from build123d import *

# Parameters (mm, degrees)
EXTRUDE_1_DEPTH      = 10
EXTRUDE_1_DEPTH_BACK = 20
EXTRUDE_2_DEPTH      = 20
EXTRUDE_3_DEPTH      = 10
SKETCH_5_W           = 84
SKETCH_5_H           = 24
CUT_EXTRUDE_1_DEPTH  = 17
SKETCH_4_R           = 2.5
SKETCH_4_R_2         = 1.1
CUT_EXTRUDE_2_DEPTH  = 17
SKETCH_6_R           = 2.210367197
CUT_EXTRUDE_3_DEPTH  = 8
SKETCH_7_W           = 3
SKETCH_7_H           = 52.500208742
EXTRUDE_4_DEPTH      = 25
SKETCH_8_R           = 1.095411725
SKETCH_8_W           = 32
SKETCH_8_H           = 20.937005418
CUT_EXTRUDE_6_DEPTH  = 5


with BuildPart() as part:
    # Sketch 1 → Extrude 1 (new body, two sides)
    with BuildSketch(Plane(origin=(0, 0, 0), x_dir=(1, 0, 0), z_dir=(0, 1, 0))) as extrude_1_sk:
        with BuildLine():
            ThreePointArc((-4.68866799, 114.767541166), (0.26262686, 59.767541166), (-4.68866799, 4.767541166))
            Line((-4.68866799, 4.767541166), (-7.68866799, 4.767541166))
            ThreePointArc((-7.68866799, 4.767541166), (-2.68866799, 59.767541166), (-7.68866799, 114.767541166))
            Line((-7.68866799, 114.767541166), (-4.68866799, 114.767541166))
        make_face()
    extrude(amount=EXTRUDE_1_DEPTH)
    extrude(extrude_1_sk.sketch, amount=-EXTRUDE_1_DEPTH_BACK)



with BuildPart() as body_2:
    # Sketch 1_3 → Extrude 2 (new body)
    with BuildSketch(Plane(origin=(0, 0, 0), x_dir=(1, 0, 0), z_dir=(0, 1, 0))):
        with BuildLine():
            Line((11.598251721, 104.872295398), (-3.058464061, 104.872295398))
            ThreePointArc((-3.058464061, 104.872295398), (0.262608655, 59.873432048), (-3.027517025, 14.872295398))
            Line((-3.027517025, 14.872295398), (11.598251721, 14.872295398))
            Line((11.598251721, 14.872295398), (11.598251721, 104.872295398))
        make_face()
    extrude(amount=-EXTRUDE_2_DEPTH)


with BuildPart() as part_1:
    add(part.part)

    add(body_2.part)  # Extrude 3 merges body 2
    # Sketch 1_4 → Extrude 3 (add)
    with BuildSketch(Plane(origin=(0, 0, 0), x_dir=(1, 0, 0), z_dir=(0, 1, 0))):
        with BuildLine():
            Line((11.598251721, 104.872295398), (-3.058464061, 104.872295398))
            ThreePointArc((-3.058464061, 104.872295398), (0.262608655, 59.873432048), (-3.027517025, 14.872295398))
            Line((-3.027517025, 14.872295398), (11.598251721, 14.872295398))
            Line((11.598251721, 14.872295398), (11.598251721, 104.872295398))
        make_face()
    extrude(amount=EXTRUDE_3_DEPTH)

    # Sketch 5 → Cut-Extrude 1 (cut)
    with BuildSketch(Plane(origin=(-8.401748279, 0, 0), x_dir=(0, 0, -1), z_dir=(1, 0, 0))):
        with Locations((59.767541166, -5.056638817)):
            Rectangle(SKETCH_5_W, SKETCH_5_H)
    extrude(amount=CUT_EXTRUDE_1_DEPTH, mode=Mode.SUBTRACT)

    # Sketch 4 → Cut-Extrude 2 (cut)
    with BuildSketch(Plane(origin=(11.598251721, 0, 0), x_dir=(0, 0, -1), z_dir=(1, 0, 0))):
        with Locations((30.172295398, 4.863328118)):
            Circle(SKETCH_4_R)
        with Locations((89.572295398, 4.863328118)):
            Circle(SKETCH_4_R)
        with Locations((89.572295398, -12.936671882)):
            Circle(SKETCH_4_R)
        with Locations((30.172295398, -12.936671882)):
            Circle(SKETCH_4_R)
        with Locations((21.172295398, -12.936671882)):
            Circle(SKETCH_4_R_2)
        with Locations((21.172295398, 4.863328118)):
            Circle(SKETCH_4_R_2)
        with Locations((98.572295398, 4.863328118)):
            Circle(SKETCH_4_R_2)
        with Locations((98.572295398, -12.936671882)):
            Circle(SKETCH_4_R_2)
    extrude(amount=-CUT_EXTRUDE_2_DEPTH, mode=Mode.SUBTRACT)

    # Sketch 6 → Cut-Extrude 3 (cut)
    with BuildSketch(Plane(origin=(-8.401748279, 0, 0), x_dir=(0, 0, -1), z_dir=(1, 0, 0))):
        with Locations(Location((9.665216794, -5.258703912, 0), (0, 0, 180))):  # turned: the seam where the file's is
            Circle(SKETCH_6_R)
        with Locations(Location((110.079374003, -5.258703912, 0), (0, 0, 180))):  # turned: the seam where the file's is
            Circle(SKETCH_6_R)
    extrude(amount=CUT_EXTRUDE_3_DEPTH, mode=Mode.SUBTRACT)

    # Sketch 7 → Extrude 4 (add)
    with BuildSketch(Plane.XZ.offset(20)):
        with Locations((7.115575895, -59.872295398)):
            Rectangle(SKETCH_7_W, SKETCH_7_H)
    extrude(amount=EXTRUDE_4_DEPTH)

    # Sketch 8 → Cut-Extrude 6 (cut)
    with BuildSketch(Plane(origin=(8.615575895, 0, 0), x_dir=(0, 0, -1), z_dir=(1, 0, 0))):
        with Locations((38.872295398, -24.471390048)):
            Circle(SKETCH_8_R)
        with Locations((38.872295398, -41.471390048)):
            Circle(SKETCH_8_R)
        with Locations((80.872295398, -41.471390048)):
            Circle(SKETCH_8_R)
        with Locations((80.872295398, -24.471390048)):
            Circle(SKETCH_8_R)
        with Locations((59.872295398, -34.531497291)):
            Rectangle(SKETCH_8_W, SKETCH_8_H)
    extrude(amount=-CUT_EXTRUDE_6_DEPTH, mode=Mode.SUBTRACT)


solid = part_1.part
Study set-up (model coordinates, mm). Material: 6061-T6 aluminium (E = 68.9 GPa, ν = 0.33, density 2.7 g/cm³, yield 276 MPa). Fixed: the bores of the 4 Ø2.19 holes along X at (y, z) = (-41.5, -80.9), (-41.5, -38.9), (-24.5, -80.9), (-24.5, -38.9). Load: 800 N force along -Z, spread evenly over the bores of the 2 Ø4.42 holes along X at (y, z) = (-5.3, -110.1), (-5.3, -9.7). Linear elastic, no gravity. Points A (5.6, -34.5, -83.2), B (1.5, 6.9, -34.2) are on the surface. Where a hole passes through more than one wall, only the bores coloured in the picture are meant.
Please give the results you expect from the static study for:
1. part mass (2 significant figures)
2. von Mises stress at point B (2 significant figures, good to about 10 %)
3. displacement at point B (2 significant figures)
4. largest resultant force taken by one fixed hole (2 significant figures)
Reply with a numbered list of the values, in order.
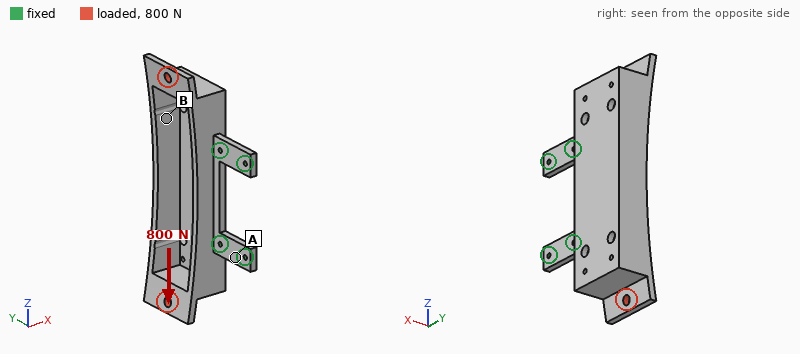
1. 54 g
2. 18 MPa
3. 0.11 mm
4. 570 N
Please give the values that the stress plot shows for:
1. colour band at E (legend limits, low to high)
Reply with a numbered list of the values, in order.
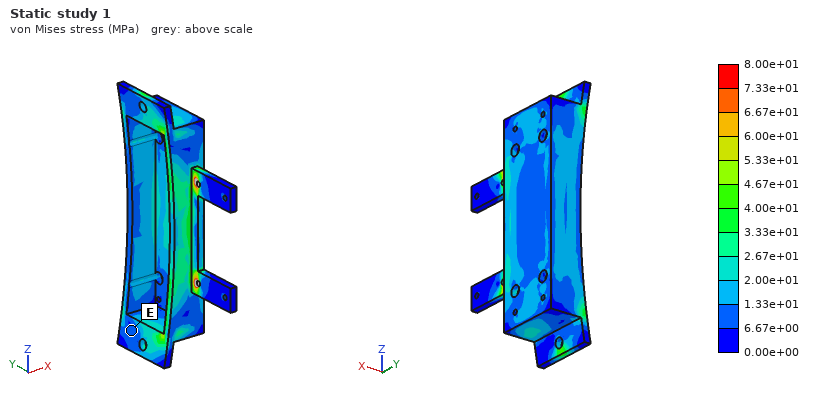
1. 6.67e+00 to 1.33e+01 MPa
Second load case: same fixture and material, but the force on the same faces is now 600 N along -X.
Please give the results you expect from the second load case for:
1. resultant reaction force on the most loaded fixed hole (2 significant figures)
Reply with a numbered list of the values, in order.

1. 370 N
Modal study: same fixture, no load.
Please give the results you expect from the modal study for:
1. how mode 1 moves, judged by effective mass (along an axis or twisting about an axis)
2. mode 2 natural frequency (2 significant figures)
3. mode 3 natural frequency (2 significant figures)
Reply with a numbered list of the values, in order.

1. along X
2. 1400 Hz
3. 4200 Hz
